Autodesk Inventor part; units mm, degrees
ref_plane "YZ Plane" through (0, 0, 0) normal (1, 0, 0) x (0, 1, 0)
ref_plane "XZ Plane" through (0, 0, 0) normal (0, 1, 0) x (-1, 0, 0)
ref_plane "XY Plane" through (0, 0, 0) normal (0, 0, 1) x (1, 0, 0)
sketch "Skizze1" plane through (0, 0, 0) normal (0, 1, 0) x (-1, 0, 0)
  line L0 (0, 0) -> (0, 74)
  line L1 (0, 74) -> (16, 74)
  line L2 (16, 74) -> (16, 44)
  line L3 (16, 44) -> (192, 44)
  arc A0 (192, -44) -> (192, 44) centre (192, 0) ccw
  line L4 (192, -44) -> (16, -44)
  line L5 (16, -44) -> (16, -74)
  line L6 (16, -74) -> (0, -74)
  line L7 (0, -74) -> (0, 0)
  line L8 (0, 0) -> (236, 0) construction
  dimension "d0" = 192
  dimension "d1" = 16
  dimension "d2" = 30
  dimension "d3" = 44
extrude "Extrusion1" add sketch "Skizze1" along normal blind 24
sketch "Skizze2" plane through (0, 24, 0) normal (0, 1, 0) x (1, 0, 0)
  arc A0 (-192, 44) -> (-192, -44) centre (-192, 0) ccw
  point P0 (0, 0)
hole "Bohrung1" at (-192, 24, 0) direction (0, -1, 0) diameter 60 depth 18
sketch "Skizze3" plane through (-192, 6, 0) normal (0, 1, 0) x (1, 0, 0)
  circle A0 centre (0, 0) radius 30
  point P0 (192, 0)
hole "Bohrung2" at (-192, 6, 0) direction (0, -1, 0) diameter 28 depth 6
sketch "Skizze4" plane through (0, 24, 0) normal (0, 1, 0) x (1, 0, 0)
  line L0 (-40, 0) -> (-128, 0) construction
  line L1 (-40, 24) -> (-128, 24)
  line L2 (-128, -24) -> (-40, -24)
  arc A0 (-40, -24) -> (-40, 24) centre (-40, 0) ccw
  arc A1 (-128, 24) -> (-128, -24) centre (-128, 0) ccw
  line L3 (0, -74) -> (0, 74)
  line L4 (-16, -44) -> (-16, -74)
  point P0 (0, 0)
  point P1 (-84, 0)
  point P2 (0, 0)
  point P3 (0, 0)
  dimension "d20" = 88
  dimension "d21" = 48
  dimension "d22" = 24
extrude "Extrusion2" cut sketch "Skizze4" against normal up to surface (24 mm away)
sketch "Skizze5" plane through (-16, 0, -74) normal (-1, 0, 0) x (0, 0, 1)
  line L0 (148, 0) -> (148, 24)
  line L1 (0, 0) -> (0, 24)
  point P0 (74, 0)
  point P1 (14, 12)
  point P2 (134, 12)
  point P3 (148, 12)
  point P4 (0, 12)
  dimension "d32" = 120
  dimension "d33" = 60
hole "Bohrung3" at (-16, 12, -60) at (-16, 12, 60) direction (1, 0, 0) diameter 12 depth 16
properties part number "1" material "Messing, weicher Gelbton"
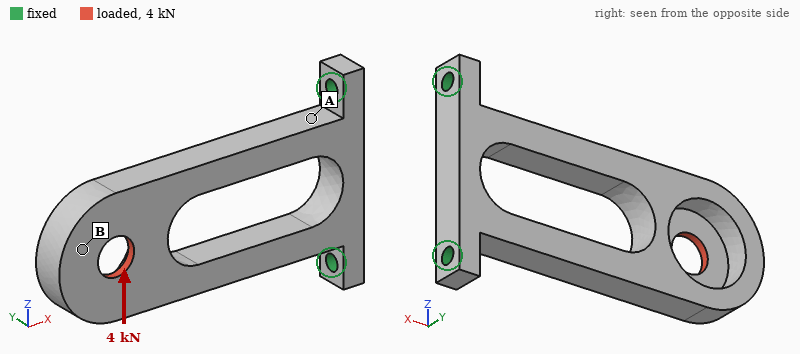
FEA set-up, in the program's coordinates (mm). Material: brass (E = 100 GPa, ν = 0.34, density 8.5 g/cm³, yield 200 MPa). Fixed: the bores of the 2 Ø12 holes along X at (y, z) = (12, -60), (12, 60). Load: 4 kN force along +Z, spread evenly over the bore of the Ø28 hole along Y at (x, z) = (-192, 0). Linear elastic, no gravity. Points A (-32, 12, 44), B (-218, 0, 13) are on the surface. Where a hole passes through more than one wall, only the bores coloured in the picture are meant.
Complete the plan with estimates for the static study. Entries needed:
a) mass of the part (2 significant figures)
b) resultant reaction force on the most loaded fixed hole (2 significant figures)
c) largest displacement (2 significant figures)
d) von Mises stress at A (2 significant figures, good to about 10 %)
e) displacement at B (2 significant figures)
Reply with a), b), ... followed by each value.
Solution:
a) 2.5 kg
b) 7.8 kN
c) 0.41 mm
d) 73 MPa
e) 0.40 mm
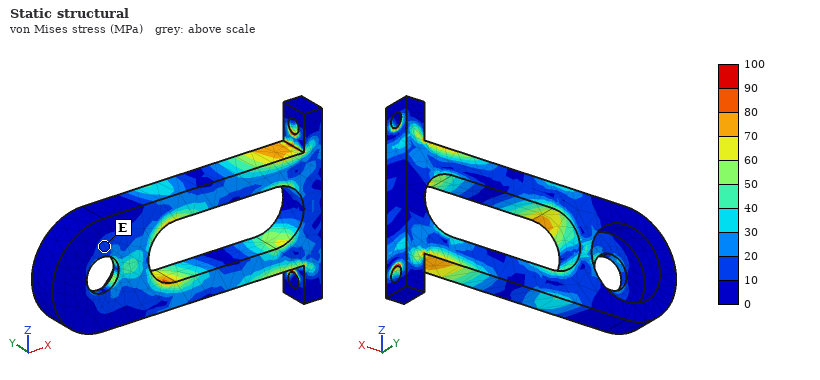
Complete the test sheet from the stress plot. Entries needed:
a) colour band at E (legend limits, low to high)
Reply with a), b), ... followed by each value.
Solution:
a) 10 to 20 MPa
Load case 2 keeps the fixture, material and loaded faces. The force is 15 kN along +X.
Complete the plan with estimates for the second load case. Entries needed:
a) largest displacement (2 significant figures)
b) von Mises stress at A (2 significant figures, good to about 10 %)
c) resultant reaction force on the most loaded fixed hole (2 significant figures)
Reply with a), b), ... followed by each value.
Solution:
a) 1.0 mm
b) 35 MPa
c) 7.7 kN
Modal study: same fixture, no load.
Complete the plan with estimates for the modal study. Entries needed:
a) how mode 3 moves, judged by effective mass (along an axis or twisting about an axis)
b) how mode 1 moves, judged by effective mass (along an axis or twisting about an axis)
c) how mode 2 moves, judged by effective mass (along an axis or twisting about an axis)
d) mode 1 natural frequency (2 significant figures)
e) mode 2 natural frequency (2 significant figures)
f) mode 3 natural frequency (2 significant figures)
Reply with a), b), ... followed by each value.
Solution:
a) twisting about X
b) along Y
c) along Z
d) 180 Hz
e) 480 Hz
f) 740 Hz
